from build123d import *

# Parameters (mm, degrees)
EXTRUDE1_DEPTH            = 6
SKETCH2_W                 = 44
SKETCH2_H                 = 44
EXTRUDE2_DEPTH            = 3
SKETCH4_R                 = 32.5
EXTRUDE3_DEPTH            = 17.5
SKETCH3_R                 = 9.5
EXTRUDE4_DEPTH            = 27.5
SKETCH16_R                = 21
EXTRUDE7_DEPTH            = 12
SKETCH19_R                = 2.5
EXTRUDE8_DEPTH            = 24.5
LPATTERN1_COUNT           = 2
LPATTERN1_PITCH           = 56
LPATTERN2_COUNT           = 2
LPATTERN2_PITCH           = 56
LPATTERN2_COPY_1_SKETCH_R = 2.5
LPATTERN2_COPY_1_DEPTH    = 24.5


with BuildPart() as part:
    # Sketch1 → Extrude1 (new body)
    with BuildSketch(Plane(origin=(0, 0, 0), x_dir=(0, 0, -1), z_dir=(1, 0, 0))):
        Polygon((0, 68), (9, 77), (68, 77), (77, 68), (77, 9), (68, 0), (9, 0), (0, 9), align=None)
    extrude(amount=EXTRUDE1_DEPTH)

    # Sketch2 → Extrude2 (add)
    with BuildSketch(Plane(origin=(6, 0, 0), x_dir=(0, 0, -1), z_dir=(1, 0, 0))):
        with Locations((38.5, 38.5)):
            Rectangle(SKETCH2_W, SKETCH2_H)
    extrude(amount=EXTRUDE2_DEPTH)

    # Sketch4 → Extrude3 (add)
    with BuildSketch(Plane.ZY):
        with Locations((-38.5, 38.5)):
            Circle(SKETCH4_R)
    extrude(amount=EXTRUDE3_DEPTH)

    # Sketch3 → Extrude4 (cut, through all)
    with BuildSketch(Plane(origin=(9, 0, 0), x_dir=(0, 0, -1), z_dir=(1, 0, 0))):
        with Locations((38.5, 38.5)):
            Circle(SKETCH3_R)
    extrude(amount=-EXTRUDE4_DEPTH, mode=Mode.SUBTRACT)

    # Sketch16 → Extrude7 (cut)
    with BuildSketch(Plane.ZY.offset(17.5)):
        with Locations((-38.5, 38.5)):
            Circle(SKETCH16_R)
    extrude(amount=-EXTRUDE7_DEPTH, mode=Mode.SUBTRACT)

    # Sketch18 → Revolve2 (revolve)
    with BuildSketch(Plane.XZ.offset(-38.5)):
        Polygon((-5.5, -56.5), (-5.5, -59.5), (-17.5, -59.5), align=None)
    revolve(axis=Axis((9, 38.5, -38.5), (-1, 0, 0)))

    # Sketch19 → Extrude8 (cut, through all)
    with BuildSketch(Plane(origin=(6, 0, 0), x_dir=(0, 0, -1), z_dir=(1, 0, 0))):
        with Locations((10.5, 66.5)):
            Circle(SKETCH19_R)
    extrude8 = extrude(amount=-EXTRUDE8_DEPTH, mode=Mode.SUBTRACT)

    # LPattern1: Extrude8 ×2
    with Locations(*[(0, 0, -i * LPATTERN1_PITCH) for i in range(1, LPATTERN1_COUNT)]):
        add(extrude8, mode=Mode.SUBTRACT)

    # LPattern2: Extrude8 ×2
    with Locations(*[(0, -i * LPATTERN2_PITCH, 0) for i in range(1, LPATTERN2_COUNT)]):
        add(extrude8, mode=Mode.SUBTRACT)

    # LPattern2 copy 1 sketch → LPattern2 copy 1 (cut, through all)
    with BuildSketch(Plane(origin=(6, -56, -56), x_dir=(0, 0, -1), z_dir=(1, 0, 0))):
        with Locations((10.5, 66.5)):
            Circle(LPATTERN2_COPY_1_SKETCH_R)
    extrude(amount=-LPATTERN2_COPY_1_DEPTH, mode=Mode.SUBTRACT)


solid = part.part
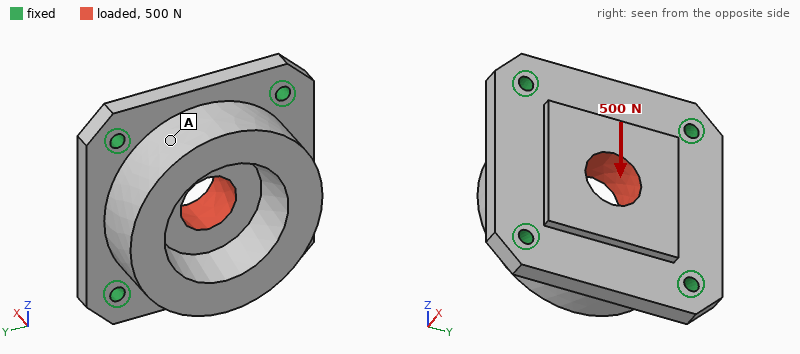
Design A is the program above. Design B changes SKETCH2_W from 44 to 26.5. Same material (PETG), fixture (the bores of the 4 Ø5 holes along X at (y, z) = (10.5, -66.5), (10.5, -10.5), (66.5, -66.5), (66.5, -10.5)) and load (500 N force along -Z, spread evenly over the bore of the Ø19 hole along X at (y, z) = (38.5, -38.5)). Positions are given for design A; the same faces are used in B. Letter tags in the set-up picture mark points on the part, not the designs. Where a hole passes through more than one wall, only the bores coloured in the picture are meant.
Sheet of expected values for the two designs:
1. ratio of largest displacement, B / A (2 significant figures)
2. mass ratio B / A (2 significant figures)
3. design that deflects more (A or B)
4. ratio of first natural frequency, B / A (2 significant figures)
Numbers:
1.2
0.97
B
1.0
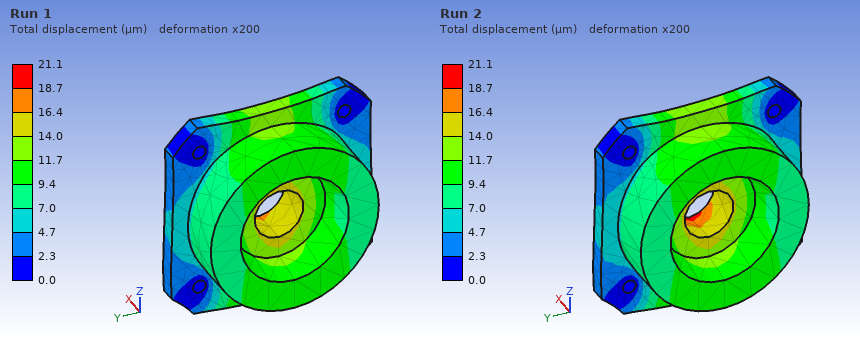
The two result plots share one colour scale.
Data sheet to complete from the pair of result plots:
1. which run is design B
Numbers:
Run 2
